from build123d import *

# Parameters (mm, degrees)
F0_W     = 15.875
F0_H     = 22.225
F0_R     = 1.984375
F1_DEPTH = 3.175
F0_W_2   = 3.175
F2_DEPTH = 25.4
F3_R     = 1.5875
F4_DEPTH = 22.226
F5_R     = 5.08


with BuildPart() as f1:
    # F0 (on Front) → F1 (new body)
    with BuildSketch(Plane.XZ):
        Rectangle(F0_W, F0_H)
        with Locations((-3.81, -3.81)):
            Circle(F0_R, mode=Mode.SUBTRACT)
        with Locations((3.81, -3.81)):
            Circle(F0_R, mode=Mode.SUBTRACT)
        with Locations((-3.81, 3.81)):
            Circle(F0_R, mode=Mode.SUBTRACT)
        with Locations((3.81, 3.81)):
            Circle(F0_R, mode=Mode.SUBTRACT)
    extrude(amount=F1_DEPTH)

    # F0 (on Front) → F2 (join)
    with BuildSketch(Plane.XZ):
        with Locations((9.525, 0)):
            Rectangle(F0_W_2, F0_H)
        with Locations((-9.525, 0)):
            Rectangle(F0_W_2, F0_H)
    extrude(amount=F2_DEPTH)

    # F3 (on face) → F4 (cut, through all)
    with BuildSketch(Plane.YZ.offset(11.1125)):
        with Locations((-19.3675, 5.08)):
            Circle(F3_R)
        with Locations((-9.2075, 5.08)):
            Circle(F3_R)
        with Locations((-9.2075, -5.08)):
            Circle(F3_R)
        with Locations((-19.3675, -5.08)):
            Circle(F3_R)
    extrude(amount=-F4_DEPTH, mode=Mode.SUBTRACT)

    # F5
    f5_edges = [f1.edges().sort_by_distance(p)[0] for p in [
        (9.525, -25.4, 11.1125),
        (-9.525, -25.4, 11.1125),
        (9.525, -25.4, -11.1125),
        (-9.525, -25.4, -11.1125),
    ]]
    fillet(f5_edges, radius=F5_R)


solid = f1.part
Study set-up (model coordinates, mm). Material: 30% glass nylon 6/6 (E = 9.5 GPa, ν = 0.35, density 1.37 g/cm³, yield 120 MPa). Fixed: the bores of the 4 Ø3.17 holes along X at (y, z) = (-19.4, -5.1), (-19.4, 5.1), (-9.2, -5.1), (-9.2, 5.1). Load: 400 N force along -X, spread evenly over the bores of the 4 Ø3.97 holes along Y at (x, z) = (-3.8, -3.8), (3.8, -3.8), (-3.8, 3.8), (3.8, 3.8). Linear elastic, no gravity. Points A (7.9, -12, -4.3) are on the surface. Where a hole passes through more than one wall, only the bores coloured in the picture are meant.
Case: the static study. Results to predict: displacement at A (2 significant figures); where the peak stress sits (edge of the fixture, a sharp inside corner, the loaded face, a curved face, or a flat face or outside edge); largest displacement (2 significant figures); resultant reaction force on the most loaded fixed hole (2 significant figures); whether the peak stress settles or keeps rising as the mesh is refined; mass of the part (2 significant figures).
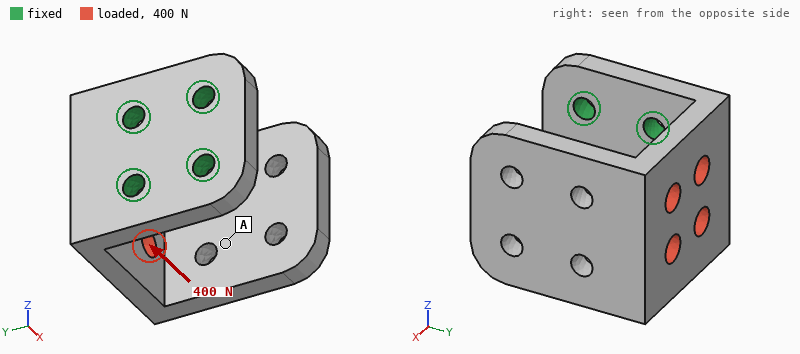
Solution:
0.32 mm
edge of the fixture
0.48 mm
230 N
keeps rising
5.9 g
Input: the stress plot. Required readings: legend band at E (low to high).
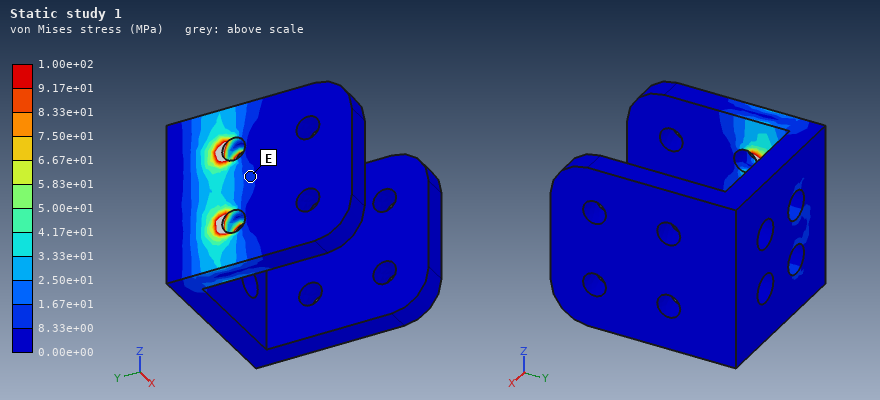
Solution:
8.33e+00 to 1.67e+01 MPa
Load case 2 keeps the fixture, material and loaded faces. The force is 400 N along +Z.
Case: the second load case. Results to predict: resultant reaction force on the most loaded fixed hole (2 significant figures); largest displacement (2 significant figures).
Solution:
390 N
0.47 mm
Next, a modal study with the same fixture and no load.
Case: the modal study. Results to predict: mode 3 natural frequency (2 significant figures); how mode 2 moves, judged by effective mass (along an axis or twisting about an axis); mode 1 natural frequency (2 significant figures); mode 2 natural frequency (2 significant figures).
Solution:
2200 Hz
along Z
810 Hz
1300 Hz
